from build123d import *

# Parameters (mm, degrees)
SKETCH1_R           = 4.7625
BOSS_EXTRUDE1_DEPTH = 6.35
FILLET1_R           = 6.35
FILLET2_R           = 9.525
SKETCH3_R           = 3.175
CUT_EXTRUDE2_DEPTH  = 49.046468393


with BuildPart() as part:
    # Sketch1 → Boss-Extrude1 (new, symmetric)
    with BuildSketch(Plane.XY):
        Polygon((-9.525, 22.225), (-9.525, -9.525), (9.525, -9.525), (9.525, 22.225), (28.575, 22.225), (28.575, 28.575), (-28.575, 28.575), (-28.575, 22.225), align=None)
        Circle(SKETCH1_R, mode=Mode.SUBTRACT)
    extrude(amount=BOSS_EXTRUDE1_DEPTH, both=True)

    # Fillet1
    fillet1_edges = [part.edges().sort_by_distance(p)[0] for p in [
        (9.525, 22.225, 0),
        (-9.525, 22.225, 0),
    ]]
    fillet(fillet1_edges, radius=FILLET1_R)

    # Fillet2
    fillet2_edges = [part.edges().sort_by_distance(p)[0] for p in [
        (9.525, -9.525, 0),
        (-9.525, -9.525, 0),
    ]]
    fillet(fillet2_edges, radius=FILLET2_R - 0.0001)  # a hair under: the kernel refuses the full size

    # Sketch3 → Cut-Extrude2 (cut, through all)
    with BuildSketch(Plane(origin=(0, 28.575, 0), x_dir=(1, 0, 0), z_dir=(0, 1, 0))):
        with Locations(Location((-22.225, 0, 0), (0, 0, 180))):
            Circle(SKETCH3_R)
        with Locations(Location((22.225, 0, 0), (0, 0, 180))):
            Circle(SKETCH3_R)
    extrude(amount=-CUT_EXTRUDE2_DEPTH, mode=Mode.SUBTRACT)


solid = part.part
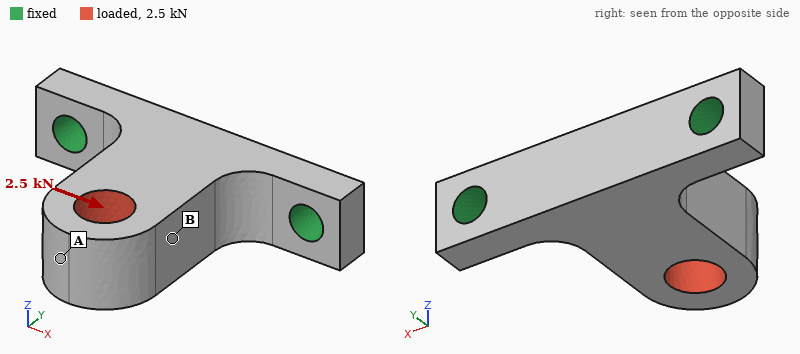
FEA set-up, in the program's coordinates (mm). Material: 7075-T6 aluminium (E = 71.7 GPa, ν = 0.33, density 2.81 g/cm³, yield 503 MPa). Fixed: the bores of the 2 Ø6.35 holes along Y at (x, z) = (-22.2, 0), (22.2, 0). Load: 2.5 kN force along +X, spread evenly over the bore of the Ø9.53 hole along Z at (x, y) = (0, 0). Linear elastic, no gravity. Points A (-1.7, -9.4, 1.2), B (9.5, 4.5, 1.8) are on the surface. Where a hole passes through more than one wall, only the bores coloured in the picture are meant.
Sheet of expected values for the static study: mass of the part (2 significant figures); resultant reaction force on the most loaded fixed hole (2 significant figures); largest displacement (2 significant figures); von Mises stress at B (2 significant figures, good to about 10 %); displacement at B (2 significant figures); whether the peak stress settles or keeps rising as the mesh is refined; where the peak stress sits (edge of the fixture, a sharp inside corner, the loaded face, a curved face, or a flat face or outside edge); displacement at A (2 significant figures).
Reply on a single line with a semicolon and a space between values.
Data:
30 g; 2.3 kN; 86 µm; 36 MPa; 50 µm; keeps rising; edge of the fixture; 86 µm
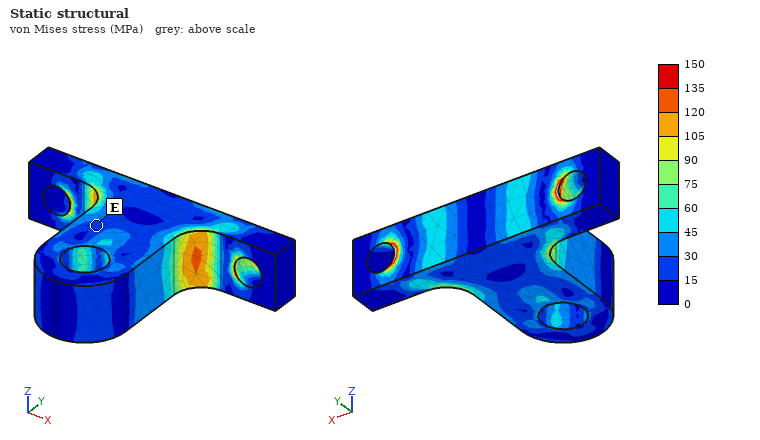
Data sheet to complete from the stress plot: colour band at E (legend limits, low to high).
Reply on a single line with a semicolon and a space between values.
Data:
15 to 30 MPa
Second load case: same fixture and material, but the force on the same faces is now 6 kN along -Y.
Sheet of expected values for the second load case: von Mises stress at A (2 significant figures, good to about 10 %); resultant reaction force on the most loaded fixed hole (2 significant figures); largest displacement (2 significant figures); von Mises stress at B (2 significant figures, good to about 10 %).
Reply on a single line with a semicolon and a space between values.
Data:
29 MPa; 3.5 kN; 50 µm; 22 MPa
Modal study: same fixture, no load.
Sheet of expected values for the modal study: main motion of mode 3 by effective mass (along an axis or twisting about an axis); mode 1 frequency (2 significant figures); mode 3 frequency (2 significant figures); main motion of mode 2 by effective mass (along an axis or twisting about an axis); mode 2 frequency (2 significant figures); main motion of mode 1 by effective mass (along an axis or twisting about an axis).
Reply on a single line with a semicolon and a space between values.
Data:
along Y; 3900 Hz; 13 kHz; along X; 10 kHz; along Z
